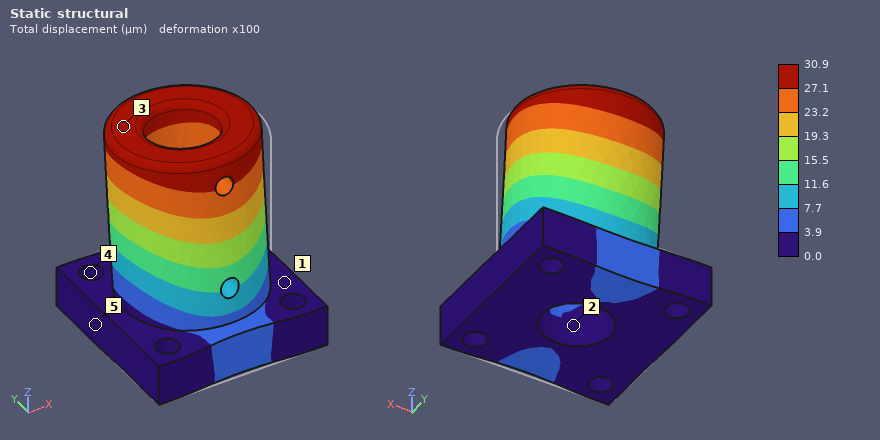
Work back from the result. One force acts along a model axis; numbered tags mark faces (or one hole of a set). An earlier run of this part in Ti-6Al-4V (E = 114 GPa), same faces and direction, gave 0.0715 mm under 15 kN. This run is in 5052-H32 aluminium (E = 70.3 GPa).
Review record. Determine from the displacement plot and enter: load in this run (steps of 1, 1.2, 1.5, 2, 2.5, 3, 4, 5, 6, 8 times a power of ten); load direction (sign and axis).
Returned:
4 kN
+Y
